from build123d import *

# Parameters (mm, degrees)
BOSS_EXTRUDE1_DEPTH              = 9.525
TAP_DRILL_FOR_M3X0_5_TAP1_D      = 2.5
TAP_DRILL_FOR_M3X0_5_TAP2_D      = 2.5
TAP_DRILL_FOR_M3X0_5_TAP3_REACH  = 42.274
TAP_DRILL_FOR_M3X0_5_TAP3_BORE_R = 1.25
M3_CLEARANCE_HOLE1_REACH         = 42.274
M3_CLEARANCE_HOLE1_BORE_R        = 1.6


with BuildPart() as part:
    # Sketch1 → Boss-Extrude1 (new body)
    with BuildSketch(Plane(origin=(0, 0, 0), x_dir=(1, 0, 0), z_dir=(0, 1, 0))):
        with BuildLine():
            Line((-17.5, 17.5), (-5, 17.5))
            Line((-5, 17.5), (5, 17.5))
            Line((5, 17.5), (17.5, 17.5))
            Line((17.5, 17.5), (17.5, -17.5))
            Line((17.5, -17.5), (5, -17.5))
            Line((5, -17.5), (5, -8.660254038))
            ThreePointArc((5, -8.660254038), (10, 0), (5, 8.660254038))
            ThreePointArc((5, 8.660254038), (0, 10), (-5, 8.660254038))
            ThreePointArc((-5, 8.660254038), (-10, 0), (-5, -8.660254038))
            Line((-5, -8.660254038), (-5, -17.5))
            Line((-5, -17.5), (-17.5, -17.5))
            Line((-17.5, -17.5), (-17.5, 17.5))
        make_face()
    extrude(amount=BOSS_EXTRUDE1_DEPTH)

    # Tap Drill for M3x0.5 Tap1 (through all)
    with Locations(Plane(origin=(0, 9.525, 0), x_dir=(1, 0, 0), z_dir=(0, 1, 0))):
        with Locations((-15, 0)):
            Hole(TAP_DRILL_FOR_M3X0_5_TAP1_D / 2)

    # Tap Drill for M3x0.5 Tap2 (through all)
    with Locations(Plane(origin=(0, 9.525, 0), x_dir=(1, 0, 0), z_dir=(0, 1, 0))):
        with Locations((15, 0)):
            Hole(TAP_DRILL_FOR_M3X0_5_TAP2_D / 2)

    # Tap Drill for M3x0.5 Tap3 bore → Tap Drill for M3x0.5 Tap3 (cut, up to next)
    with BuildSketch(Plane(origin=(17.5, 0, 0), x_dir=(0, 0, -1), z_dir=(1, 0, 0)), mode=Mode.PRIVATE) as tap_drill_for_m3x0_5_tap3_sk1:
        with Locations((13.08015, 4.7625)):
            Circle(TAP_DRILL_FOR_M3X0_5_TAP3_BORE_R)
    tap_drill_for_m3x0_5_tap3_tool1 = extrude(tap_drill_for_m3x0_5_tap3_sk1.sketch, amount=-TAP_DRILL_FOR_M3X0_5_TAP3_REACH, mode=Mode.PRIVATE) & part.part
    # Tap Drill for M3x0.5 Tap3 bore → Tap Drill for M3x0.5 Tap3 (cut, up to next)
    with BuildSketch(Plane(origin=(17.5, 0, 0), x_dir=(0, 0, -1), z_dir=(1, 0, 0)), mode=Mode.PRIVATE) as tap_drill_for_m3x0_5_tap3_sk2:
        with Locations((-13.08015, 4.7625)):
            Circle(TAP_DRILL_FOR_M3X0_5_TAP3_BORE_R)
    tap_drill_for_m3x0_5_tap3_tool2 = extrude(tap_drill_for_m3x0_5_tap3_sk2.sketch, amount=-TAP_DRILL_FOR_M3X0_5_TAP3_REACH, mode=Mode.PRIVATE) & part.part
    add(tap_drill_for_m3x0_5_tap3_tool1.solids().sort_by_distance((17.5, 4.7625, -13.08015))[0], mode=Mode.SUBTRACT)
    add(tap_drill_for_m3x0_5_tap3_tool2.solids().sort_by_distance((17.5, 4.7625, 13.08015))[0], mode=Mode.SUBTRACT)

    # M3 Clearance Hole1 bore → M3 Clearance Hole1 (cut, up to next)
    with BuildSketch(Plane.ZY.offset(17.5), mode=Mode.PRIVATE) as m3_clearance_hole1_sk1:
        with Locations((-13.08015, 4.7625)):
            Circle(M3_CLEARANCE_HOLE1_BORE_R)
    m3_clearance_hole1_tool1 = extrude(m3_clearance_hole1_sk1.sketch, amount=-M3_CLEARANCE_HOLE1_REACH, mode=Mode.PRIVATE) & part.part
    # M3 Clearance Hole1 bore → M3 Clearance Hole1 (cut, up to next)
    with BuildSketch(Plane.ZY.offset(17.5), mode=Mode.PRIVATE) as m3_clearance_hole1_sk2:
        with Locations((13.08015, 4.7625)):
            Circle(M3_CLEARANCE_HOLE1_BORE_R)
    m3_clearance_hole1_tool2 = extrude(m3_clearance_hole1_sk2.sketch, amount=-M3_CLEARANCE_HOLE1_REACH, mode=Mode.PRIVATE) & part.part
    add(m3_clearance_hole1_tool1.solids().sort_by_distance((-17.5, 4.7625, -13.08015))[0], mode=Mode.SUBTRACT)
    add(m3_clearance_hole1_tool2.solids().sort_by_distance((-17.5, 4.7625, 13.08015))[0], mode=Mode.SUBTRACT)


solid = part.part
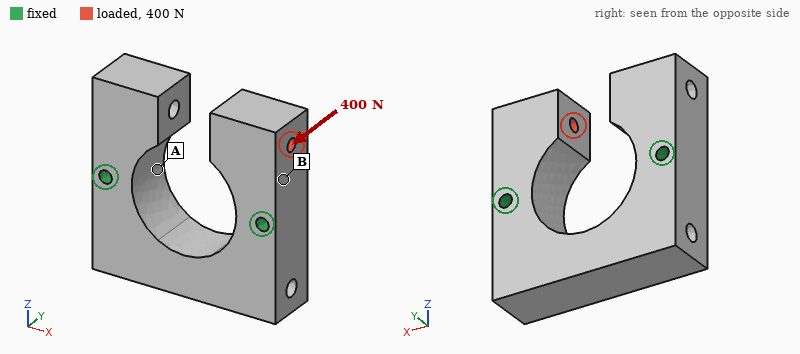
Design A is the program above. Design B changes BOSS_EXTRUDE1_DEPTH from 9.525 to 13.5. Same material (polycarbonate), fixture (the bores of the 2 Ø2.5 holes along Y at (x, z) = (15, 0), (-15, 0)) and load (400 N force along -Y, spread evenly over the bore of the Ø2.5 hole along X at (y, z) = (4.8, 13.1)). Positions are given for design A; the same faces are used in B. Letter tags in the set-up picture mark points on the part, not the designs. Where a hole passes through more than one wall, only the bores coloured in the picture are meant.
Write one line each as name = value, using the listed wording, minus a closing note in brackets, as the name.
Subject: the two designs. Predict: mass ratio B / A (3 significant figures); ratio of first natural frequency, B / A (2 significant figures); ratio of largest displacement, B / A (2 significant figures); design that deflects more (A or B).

mass ratio B / A = 1.44
ratio of first natural frequency, B / A = 1.00
ratio of largest displacement, B / A = 0.42
design that deflects more = A
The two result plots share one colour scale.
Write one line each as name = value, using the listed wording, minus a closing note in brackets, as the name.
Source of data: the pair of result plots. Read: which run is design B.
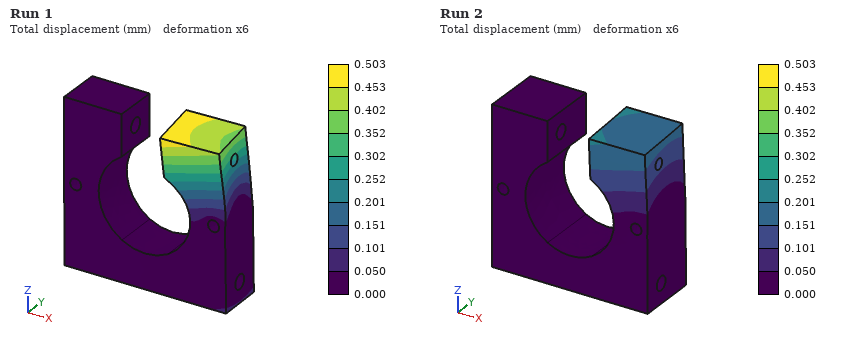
which run is design B = Run 2
